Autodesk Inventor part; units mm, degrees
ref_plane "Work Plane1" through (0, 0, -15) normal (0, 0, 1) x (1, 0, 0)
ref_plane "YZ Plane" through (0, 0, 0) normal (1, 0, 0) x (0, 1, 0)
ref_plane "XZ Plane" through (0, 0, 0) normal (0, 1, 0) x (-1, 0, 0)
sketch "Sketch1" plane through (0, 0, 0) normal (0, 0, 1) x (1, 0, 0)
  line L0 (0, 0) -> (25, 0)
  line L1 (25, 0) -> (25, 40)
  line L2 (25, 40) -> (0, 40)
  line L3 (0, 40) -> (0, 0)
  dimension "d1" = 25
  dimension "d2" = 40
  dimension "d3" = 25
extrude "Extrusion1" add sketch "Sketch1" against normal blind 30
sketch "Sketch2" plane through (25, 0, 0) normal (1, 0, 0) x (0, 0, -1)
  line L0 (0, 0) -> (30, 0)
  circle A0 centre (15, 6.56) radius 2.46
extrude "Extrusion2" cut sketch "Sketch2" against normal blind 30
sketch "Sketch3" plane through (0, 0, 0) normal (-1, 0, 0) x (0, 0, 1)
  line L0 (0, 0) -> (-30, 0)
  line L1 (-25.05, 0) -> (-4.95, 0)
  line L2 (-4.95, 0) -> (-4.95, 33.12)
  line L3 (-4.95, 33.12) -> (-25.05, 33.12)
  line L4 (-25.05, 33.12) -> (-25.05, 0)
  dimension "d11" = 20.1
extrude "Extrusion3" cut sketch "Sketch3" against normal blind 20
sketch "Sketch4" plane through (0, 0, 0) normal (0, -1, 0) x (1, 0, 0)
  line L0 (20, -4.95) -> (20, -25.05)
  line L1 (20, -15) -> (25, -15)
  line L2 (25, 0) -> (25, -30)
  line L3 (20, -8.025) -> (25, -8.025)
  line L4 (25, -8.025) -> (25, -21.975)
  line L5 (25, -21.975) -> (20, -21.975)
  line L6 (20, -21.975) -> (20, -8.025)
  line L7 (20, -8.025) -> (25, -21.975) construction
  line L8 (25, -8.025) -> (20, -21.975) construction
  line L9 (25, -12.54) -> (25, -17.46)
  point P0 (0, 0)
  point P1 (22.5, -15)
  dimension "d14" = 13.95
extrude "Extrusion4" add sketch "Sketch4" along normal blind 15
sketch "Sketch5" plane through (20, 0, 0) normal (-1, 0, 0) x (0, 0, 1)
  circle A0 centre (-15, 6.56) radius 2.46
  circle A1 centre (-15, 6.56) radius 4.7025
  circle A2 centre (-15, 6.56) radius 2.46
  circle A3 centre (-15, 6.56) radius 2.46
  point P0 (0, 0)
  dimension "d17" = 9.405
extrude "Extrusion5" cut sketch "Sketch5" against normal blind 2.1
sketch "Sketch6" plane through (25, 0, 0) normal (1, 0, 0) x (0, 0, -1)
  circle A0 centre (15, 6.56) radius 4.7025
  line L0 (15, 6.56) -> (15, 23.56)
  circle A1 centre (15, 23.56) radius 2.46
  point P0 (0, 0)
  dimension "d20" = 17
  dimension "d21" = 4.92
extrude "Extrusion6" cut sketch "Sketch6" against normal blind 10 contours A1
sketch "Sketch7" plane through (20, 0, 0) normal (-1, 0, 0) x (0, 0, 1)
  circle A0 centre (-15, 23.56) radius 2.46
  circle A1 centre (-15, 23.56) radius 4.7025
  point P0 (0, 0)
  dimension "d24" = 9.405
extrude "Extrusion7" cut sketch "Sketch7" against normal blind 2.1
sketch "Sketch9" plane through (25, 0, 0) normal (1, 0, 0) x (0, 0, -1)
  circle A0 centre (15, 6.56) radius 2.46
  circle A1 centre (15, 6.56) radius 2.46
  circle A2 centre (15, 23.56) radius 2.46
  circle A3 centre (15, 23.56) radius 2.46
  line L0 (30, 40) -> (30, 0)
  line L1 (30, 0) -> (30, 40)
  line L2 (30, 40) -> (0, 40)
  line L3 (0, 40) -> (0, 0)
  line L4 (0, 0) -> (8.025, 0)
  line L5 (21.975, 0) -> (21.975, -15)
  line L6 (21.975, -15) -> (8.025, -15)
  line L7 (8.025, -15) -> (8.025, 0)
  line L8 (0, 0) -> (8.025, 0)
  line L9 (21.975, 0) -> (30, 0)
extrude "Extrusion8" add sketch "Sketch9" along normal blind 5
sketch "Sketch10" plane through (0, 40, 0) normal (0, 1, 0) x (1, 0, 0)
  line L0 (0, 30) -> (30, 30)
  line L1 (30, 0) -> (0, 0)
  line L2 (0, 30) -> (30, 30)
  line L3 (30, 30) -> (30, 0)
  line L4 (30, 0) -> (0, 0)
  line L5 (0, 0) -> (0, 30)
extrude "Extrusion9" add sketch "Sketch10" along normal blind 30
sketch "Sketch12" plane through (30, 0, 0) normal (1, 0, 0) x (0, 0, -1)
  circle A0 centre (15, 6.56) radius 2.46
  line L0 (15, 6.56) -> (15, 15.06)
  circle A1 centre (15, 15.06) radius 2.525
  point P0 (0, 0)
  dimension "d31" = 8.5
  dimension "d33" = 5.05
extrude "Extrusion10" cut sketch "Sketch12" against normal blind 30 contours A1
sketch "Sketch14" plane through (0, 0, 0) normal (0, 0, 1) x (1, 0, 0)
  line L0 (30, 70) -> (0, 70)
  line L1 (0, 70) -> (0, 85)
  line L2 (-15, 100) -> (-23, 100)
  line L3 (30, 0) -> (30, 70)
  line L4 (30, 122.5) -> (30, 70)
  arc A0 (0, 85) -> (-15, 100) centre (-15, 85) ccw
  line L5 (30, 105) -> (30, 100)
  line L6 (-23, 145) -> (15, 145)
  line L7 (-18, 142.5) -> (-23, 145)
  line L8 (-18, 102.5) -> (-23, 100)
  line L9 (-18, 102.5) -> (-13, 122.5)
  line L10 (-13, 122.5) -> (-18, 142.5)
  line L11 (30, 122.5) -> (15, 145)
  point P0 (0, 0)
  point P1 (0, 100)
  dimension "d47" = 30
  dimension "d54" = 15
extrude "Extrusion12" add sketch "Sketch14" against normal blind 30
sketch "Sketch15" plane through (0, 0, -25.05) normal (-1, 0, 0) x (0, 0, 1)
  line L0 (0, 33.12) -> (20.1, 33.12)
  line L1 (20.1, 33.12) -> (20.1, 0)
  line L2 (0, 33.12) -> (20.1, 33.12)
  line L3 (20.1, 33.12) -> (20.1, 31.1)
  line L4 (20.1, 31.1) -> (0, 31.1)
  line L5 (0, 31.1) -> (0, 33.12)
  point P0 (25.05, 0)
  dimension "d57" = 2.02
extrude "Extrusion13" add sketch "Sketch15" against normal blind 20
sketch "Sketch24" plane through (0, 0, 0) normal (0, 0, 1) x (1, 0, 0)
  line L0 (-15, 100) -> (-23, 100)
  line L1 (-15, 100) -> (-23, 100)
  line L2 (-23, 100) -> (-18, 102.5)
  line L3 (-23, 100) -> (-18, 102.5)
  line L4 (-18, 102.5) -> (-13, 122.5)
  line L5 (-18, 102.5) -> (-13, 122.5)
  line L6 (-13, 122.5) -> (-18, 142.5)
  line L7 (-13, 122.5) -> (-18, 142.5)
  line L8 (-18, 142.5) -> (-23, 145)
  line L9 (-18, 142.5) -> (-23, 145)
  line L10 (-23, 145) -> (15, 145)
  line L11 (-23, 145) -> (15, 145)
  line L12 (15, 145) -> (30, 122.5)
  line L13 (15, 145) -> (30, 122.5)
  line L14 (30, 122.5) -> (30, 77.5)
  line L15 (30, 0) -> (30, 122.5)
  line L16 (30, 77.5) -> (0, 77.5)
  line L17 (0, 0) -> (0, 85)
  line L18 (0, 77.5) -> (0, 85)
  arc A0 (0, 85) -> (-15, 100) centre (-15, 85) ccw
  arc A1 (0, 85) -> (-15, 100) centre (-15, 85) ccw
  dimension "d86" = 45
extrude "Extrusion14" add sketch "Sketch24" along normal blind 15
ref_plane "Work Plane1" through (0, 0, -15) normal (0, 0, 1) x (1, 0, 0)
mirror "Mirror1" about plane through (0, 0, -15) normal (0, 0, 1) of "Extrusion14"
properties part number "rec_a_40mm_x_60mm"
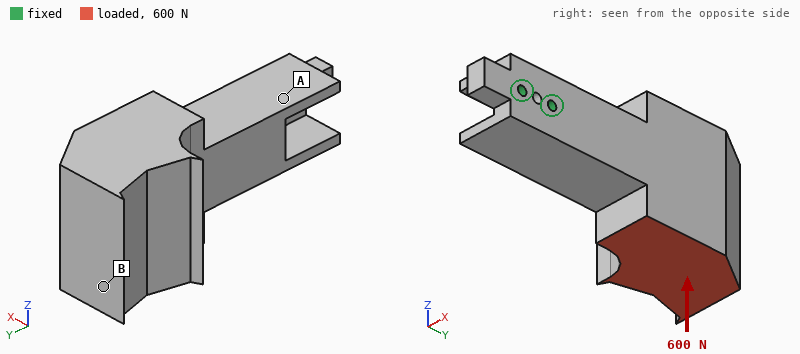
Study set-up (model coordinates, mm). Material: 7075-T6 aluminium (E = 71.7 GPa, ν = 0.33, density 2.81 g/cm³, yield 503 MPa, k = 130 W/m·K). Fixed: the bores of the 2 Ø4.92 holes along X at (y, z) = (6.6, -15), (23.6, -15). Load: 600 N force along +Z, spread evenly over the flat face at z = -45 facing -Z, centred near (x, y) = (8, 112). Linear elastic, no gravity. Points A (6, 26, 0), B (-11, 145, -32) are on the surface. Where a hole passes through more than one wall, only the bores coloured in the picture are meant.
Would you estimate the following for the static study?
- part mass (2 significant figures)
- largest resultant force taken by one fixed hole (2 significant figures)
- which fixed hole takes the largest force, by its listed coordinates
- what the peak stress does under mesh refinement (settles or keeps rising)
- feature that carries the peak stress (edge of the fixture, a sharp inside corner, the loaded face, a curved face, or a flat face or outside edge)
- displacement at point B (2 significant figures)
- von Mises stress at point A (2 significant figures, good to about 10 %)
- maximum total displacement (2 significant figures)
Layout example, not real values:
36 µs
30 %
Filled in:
610 g
2.9 kN
(23.6, -15)
keeps rising
edge of the fixture
0.14 mm
11 MPa
0.15 mm
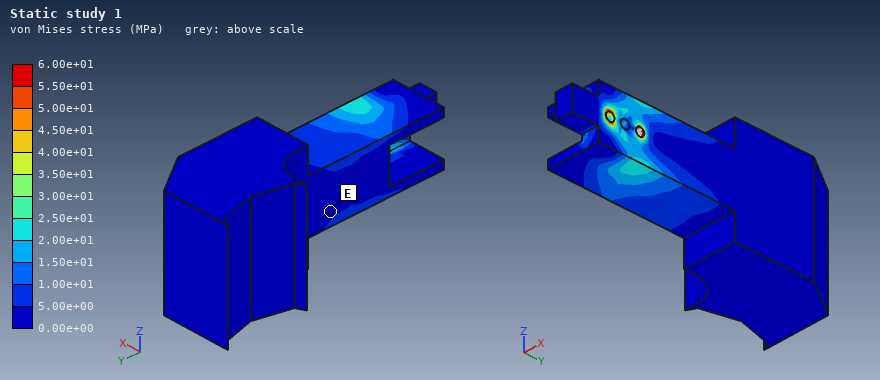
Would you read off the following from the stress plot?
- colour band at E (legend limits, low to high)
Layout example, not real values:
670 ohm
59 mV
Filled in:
0.00e+00 to 5.00e+00 MPa
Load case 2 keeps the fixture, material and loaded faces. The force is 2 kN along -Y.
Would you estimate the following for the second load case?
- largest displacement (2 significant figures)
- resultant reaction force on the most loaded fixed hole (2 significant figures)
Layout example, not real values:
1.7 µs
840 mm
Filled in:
0.22 mm
3.2 kN
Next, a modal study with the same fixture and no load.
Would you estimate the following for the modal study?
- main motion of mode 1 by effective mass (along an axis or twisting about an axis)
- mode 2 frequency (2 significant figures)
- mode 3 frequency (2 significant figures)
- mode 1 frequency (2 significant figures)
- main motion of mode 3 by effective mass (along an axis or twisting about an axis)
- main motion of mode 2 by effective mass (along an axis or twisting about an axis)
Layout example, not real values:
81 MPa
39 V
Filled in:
along X
560 Hz
1400 Hz
490 Hz
twisting about Y
along Z
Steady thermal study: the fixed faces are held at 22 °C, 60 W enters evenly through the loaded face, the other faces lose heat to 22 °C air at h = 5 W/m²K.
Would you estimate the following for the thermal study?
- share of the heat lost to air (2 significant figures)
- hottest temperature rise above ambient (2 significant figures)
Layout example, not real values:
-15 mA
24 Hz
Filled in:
7.7 %
52 K
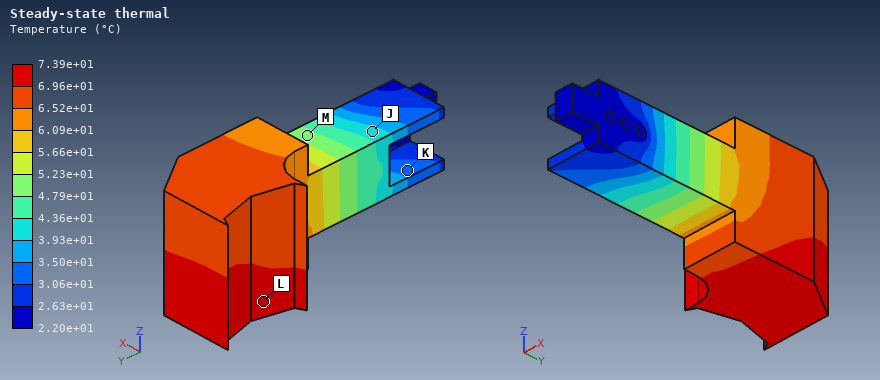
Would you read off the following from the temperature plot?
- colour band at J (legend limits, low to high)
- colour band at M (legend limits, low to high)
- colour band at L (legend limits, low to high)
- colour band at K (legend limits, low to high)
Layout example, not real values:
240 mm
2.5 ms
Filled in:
3.93e+01 to 4.36e+01 °C
4.79e+01 to 5.23e+01 °C
6.96e+01 to 7.39e+01 °C
3.06e+01 to 3.50e+01 °C
